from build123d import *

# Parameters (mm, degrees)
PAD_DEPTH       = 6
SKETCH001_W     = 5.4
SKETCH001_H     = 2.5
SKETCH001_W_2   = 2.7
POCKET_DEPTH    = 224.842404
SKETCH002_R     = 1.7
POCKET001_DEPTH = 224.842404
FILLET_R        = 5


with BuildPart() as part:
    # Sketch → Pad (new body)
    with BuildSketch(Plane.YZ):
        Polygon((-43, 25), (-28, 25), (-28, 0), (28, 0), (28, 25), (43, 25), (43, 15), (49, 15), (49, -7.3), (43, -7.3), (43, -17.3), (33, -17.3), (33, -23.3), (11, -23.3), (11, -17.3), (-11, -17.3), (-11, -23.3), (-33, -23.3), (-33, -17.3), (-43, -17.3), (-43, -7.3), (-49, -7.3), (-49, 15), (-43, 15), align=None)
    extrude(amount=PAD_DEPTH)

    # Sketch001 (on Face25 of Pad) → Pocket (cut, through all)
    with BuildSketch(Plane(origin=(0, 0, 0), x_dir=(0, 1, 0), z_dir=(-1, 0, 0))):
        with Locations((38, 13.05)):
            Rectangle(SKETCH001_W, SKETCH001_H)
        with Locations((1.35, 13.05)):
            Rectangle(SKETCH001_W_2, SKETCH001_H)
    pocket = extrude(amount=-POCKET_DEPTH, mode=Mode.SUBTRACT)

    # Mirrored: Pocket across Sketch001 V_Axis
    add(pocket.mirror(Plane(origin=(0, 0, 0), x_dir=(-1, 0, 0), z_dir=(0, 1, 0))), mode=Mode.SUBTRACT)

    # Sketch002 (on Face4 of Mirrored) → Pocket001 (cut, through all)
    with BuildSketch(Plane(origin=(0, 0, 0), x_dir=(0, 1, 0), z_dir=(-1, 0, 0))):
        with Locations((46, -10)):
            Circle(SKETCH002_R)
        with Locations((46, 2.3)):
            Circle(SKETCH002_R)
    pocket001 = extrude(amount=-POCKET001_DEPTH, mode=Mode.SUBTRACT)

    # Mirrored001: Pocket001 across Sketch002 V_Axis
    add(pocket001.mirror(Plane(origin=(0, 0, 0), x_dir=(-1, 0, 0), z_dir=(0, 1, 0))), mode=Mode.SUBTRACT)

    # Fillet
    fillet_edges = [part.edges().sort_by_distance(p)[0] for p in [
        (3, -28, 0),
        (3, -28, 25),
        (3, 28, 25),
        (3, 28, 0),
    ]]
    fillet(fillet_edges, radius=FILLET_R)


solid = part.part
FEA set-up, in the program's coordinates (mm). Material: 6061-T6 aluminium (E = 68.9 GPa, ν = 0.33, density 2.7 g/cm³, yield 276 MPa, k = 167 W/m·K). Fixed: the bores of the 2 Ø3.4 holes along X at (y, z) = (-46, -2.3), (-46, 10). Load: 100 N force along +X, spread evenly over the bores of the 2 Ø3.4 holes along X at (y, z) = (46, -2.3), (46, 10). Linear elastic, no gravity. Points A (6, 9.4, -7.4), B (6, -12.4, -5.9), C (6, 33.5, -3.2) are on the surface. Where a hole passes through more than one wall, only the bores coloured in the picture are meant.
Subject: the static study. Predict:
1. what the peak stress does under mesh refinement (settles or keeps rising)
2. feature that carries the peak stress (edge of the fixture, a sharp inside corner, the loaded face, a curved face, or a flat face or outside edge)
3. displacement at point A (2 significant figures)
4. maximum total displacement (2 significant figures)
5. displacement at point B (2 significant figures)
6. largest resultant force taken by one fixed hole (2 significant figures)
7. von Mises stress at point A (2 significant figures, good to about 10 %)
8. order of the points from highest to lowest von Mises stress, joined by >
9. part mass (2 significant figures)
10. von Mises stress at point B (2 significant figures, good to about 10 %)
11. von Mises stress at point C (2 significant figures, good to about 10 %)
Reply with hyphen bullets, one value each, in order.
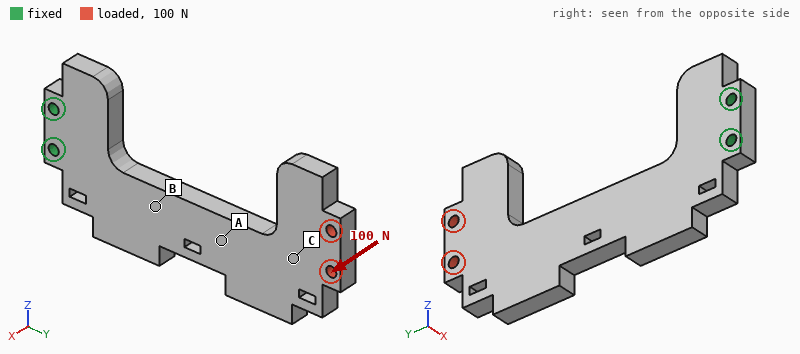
- keeps rising
- edge of the fixture
- 0.47 mm
- 1.2 mm
- 0.19 mm
- 52 N
- 37 MPa
- B > A > C
- 44 g
- 55 MPa
- 13 MPa
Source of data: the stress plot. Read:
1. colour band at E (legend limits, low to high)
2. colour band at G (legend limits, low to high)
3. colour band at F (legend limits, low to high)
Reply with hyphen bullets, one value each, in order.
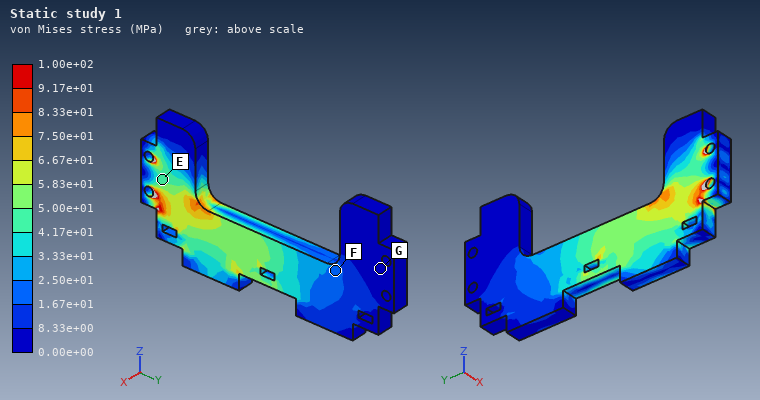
- 4.17e+01 to 5.00e+01 MPa
- 0.00e+00 to 8.33e+00 MPa
- 1.67e+01 to 2.50e+01 MPa
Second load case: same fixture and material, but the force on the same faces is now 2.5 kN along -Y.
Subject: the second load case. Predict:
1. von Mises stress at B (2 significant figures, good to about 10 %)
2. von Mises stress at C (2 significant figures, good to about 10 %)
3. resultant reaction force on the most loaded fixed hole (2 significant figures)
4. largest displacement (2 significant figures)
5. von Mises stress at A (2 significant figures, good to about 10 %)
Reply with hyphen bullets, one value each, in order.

- 57 MPa
- 43 MPa
- 1.3 kN
- 0.61 mm
- 44 MPa
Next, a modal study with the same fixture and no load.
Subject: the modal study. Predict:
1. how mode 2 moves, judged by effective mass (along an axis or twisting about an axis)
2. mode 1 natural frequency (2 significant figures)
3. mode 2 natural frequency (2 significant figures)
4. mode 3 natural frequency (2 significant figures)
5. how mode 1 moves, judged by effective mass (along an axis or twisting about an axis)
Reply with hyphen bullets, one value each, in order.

- along Z
- 430 Hz
- 1200 Hz
- 1700 Hz
- along X
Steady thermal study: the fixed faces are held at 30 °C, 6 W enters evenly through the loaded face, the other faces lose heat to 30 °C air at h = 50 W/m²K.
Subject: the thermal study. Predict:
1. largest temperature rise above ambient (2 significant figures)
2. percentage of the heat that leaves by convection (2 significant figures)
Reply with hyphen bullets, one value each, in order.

- 19 K
- 52 %
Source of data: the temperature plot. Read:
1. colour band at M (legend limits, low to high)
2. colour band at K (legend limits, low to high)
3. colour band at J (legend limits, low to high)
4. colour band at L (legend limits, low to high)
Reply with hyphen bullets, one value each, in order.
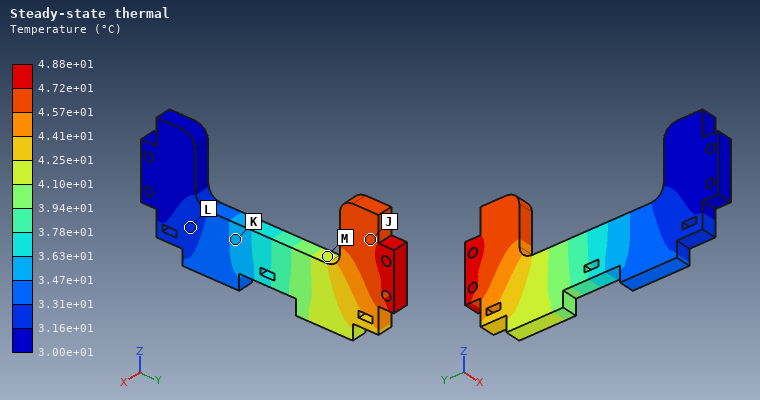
- 4.10e+01 to 4.25e+01 °C
- 3.47e+01 to 3.63e+01 °C
- 4.57e+01 to 4.72e+01 °C
- 3.16e+01 to 3.31e+01 °C
